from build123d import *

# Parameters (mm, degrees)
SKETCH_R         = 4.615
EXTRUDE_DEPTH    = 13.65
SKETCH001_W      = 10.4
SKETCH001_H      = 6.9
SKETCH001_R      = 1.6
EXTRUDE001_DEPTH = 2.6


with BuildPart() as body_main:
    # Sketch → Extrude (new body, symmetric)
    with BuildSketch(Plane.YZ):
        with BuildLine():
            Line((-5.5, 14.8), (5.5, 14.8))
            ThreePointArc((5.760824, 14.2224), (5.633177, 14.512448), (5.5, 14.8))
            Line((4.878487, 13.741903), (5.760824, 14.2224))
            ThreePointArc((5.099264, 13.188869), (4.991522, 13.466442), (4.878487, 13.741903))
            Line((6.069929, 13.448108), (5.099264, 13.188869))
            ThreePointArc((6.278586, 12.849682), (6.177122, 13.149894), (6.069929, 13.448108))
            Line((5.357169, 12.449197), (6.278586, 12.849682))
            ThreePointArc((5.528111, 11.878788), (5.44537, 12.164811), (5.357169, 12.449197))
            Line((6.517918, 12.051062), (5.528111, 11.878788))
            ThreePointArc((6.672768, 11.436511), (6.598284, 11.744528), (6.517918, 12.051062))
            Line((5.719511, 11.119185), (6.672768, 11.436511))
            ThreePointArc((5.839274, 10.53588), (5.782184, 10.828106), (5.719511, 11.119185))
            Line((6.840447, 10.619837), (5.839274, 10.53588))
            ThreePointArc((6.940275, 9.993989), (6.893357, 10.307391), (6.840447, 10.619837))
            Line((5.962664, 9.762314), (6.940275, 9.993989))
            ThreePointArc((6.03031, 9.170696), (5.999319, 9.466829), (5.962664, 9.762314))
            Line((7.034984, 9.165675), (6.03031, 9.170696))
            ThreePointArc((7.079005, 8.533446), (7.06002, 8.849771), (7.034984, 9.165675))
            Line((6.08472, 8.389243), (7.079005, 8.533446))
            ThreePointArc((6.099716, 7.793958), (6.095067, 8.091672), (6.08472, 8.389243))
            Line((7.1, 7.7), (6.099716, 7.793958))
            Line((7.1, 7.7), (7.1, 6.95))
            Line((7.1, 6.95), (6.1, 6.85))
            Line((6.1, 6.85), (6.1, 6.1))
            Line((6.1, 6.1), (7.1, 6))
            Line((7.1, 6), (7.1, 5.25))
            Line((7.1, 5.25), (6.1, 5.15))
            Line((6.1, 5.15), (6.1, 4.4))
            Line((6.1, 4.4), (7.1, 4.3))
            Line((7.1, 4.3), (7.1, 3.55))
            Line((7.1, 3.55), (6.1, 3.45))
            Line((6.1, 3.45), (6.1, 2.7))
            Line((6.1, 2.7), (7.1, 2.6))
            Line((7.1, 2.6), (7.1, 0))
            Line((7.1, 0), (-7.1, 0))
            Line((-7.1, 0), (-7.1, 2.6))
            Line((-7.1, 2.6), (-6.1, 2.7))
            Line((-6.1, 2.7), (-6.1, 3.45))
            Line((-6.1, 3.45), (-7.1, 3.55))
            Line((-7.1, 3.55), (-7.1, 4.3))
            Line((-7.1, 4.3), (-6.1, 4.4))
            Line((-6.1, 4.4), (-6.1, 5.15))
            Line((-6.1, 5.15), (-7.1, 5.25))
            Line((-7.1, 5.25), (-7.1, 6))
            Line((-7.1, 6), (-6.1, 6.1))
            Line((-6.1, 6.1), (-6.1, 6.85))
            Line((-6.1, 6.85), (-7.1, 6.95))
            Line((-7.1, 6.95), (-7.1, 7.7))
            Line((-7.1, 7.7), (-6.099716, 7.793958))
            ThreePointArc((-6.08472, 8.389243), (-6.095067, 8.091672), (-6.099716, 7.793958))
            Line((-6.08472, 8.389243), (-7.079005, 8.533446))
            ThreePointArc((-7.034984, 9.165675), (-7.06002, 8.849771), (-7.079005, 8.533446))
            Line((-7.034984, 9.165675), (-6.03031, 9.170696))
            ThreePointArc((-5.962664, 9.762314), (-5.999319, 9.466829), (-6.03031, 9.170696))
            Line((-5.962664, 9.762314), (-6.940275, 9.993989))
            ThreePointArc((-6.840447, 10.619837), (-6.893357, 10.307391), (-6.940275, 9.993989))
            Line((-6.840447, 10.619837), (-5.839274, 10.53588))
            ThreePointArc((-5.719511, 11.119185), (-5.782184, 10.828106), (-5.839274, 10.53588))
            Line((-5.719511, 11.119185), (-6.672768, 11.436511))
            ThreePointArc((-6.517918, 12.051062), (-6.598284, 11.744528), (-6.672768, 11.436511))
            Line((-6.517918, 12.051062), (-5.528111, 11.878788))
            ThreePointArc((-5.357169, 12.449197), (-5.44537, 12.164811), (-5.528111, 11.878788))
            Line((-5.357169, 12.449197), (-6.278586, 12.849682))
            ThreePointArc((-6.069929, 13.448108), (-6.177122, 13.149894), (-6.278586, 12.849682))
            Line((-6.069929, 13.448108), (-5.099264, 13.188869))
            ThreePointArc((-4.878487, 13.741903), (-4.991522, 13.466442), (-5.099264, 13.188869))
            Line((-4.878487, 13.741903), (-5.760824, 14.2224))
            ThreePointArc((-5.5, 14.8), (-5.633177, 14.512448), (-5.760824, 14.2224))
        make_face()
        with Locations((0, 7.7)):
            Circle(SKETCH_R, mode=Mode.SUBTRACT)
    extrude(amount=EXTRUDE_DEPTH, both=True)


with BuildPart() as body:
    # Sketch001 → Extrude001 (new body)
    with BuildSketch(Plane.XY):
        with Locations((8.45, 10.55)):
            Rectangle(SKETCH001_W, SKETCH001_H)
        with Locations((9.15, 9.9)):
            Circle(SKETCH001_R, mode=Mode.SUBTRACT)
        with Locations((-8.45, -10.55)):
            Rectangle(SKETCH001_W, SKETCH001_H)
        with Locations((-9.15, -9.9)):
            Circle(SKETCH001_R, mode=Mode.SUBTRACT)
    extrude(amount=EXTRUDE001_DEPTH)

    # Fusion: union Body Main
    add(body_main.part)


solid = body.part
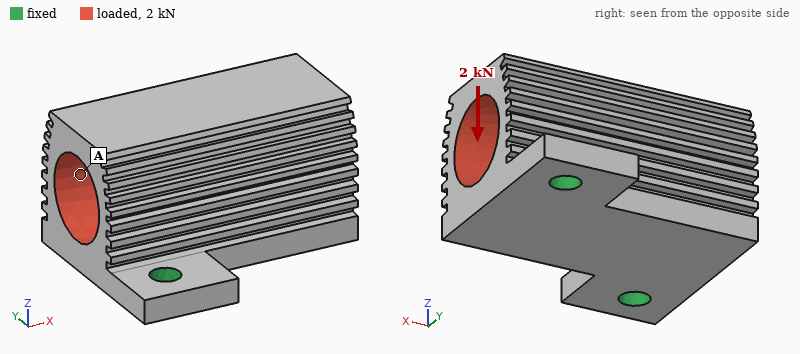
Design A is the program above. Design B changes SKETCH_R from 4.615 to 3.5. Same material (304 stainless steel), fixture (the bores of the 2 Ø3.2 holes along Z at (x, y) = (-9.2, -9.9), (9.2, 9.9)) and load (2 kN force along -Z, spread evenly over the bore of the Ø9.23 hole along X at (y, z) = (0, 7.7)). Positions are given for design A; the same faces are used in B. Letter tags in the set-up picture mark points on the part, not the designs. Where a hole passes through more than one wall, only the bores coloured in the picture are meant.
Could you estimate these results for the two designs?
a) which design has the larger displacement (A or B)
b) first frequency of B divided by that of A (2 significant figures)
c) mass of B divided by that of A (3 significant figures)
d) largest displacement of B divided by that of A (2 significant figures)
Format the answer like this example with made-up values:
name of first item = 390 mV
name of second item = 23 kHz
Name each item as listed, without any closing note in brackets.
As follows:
which design has the larger displacement = A
first frequency of B divided by that of A = 0.94
mass of B divided by that of A = 1.21
largest displacement of B divided by that of A = 0.78
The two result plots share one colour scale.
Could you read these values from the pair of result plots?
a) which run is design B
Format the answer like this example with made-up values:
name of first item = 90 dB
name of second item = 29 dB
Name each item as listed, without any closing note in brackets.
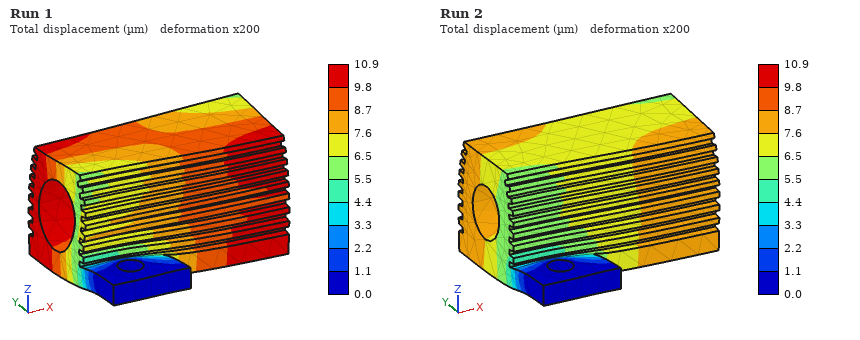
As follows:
which run is design B = Run 2
